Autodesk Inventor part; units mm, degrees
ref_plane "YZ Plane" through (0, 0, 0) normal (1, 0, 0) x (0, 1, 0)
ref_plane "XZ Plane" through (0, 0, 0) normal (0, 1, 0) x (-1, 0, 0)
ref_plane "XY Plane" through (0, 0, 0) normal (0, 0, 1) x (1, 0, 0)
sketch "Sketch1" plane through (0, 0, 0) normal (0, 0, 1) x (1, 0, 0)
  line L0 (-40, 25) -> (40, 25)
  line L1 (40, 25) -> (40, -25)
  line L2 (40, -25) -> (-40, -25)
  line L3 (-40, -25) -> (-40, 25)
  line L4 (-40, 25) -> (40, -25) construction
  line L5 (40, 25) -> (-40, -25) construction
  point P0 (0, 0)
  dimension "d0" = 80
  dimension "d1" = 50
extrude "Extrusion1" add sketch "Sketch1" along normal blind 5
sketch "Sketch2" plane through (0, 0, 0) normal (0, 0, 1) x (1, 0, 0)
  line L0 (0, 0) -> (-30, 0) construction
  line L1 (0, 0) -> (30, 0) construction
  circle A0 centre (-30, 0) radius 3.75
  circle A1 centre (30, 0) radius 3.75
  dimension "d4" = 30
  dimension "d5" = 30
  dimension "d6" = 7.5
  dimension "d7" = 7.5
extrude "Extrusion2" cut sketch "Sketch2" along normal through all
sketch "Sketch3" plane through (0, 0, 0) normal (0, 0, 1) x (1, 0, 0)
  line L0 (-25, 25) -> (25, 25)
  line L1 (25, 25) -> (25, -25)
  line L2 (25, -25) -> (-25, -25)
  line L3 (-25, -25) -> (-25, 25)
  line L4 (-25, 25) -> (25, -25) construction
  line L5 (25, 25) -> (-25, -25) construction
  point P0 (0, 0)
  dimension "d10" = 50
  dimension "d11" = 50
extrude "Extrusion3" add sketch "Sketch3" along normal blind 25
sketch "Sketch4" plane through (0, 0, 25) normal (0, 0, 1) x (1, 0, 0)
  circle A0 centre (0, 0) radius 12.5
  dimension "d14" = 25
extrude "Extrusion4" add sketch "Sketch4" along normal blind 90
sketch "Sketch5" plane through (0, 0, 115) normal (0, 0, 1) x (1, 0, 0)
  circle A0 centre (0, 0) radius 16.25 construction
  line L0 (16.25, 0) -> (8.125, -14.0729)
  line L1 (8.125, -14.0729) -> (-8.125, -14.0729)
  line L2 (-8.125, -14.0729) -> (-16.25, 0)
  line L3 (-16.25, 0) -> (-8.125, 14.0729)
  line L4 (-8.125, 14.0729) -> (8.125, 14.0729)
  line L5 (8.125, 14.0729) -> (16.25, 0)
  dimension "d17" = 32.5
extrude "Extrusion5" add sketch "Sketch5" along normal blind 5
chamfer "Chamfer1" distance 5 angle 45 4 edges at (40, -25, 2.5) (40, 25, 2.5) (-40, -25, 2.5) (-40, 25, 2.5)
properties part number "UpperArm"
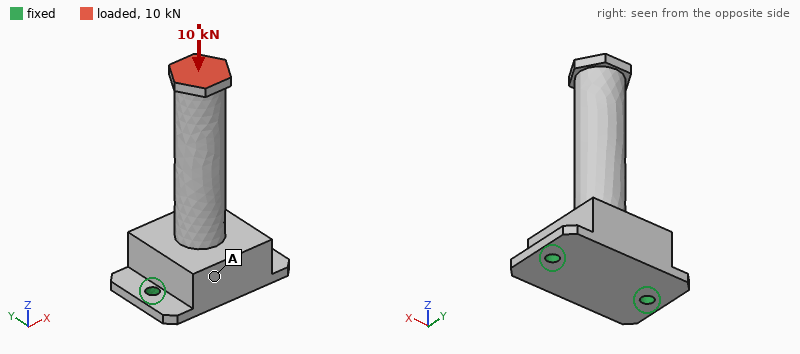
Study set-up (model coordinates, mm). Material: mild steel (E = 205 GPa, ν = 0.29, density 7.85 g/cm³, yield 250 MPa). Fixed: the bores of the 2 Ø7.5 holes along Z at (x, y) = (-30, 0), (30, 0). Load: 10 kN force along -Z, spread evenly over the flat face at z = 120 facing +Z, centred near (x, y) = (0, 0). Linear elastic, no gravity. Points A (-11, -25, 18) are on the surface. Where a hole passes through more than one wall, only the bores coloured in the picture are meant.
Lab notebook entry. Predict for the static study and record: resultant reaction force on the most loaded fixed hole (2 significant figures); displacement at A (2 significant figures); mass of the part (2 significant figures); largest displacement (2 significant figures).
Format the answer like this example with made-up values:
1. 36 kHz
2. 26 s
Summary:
1. 5.7 kN
2. 7.6 µm
3. 920 g
4. 18 µm
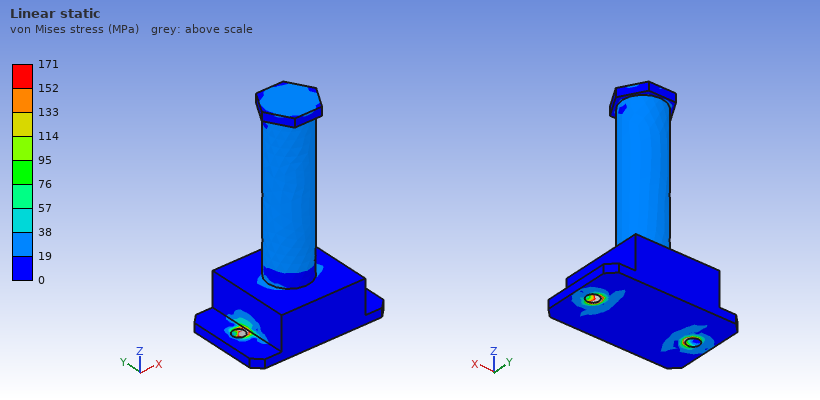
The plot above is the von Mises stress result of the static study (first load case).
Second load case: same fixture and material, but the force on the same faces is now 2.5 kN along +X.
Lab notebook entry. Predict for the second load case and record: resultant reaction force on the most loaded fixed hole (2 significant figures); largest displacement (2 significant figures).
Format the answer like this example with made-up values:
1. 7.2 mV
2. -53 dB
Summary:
1. 5.7 kN
2. 0.26 mm
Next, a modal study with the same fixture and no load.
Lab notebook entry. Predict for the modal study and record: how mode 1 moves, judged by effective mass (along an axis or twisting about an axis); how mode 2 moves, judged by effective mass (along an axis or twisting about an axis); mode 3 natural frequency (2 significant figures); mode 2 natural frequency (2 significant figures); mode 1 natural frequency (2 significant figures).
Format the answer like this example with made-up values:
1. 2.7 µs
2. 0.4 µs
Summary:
1. along Y
2. along X
3. 4500 Hz
4. 1500 Hz
5. 680 Hz
